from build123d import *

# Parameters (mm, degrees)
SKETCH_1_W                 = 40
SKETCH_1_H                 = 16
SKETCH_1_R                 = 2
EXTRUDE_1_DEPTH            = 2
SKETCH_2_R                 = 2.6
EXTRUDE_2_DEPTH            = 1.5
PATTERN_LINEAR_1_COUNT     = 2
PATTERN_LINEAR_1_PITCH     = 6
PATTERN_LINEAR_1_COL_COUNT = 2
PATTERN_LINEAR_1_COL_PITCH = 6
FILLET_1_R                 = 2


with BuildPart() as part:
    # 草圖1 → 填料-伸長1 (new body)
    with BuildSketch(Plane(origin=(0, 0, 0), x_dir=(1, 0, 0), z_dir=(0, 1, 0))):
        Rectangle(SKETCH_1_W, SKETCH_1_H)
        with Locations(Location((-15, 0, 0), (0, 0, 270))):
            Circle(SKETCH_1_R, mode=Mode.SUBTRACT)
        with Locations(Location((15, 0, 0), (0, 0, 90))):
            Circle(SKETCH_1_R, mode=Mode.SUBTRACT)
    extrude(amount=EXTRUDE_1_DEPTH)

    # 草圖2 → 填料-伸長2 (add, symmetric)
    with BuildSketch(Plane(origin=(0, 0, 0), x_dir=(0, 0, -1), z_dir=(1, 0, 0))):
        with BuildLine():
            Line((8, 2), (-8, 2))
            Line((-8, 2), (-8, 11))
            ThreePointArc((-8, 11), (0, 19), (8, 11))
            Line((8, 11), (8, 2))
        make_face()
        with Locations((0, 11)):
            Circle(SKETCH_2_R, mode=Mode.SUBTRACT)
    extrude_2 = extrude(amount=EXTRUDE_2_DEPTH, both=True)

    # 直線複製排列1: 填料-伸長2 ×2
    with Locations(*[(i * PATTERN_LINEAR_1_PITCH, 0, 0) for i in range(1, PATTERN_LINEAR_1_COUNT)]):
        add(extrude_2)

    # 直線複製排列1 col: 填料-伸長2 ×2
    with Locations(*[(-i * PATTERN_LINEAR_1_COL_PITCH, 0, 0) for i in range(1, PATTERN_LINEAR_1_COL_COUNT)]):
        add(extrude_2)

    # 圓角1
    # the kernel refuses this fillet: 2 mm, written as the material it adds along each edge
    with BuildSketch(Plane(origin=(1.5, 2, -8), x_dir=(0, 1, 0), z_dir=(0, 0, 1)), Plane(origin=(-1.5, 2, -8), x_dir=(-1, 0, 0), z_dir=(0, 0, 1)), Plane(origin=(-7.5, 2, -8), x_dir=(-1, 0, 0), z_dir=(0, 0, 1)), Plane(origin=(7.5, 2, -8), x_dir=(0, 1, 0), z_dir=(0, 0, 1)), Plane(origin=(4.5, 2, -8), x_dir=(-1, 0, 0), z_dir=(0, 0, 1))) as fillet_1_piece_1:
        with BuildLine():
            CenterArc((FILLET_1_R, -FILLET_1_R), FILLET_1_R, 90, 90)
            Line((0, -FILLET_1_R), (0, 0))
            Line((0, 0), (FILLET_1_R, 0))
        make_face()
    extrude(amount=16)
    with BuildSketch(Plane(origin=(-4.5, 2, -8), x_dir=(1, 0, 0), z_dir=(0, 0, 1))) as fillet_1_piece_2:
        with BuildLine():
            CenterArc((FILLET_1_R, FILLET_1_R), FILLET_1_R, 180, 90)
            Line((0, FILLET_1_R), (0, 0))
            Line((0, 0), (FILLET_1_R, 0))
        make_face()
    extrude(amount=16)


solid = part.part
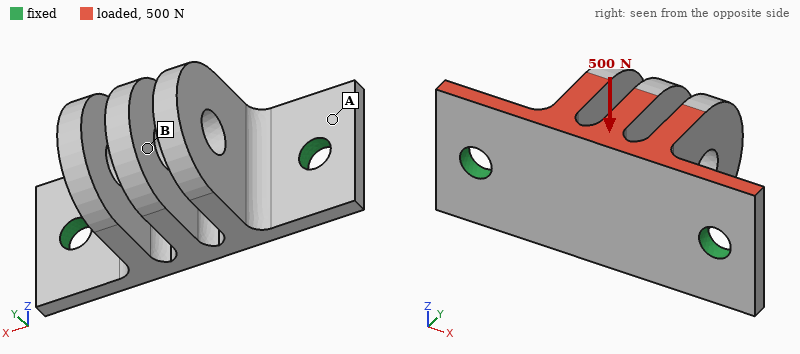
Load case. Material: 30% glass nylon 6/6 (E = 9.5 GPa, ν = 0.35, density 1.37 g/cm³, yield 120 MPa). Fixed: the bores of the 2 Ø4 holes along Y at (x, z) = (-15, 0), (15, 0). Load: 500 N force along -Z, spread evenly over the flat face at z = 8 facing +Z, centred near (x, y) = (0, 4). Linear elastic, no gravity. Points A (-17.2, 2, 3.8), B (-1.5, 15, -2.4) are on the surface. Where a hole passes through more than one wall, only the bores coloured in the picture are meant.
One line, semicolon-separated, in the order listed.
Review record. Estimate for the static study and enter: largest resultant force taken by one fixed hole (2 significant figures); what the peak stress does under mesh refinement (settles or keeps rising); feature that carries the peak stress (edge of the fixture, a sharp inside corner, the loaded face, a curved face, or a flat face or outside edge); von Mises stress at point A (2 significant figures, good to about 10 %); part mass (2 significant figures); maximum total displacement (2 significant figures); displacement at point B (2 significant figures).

250 N; keeps rising; edge of the fixture; 20 MPa; 4.5 g; 0.42 mm; 0.34 mm
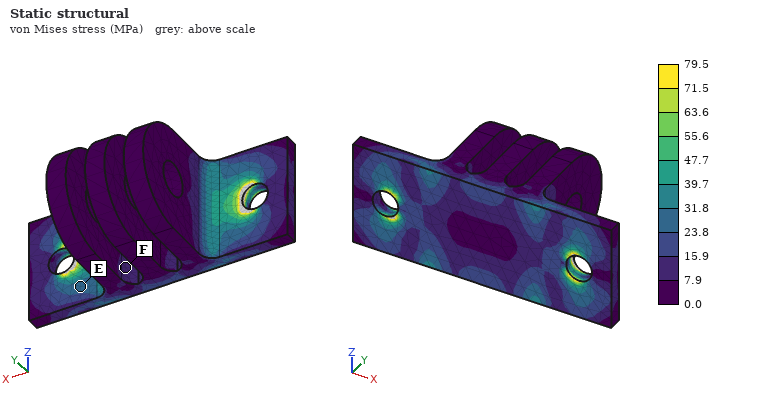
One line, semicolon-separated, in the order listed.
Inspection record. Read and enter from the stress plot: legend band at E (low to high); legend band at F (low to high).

23.8 to 31.8 MPa; 7.9 to 15.9 MPa
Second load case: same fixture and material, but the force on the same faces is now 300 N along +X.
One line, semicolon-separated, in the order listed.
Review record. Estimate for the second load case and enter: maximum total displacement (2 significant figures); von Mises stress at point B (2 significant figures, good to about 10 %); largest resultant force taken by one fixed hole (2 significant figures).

63 µm; 2.3 MPa; 170 N
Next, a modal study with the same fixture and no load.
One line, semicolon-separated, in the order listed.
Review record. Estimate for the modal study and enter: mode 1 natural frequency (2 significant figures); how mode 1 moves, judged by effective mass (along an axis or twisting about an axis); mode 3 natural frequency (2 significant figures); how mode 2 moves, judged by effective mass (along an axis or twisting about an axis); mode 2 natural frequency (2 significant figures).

2200 Hz; along Z; 4000 Hz; along Y; 2700 Hz
